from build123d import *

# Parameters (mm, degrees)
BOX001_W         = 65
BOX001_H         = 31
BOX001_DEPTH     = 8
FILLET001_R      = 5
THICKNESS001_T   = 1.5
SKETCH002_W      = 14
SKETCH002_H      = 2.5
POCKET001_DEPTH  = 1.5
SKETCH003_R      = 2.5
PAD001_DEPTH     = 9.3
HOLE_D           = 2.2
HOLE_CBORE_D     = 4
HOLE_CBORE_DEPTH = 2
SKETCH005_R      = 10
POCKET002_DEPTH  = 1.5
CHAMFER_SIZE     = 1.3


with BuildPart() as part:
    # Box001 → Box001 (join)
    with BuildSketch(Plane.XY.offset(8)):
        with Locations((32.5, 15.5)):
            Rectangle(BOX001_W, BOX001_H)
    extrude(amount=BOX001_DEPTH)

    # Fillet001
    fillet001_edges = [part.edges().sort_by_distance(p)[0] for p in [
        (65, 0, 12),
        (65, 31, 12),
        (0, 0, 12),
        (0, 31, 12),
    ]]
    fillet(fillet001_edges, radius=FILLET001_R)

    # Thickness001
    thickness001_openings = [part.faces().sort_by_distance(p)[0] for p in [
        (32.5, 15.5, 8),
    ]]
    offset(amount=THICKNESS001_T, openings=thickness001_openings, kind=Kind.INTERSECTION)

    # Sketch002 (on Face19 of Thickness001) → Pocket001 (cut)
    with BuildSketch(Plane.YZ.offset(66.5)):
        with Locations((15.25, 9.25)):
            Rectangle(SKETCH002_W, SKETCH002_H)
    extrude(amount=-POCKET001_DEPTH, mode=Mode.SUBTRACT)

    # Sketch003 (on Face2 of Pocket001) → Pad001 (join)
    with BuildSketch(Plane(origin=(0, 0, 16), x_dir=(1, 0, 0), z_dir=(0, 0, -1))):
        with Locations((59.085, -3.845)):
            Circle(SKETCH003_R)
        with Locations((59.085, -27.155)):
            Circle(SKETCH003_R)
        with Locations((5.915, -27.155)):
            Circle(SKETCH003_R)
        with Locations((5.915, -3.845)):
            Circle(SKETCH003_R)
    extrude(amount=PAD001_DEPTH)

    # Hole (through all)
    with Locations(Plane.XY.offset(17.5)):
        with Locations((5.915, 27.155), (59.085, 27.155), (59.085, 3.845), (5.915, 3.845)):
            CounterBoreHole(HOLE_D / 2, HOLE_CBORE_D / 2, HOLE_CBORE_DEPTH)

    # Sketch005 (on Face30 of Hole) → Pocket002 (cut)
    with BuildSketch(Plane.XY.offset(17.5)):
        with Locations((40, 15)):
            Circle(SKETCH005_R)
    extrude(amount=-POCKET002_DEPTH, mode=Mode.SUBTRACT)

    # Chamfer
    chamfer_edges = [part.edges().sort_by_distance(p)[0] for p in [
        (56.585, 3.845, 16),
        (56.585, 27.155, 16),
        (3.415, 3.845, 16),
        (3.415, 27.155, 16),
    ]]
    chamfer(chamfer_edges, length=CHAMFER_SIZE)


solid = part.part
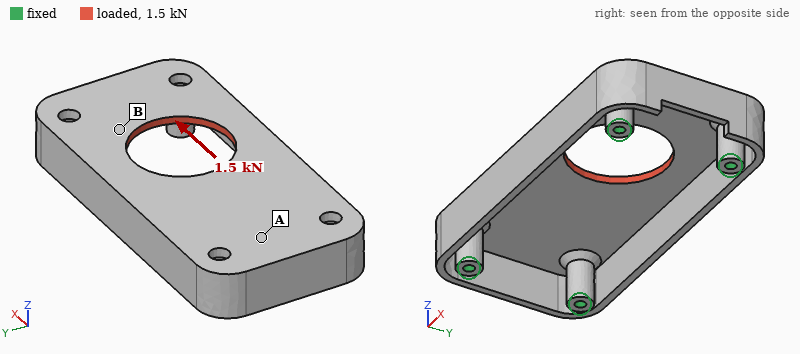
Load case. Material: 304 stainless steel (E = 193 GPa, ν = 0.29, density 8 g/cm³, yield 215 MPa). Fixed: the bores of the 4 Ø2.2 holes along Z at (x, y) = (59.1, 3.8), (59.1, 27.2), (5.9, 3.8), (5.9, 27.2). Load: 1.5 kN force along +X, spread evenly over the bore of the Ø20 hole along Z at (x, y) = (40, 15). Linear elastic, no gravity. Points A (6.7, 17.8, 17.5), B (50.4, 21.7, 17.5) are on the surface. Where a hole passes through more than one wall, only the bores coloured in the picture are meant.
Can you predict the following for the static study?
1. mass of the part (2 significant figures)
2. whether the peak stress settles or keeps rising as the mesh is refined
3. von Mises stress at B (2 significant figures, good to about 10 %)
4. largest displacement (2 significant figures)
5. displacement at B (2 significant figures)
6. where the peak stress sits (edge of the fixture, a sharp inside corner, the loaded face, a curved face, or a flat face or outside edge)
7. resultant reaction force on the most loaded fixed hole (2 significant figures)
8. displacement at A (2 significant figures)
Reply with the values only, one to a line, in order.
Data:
46 g
keeps rising
20 MPa
5.0 µm
4.0 µm
edge of the fixture
430 N
1.6 µm
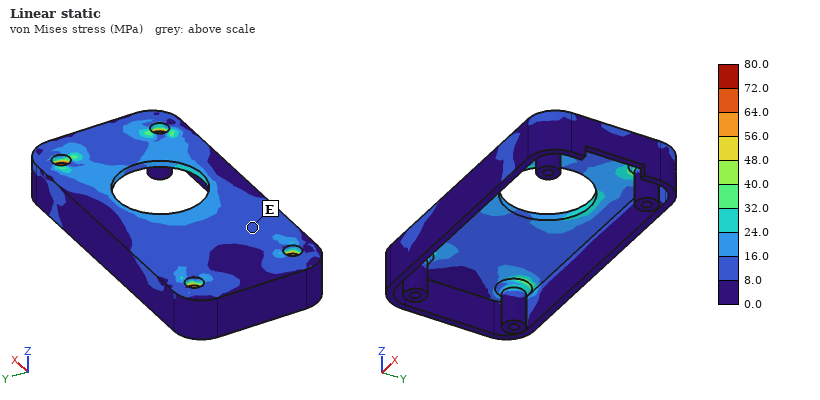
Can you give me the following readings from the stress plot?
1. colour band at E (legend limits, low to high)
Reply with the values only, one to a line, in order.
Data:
8.0 to 16.0 MPa
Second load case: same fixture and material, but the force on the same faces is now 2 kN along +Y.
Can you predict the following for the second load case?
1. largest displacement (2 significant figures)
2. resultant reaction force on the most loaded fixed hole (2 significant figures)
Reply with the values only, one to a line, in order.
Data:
14 µm
590 N
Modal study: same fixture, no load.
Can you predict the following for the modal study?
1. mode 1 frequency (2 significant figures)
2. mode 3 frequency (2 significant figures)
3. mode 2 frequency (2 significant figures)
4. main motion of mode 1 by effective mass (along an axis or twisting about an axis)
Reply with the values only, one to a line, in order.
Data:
5200 Hz
7700 Hz
7600 Hz
along Z
